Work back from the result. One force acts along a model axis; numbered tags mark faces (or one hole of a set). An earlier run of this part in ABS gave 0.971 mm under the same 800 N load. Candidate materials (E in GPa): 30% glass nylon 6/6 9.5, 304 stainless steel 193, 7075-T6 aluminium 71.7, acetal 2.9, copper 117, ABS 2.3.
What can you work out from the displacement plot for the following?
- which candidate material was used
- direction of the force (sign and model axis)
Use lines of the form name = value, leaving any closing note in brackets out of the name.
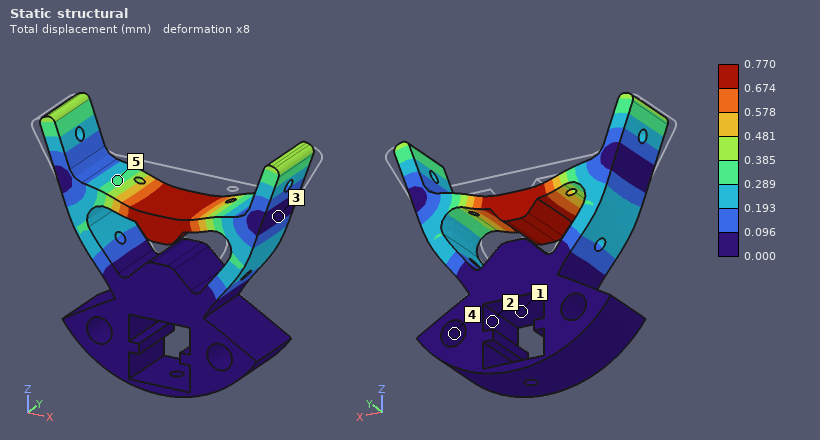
which candidate material was used = acetal
direction of the force = -Z
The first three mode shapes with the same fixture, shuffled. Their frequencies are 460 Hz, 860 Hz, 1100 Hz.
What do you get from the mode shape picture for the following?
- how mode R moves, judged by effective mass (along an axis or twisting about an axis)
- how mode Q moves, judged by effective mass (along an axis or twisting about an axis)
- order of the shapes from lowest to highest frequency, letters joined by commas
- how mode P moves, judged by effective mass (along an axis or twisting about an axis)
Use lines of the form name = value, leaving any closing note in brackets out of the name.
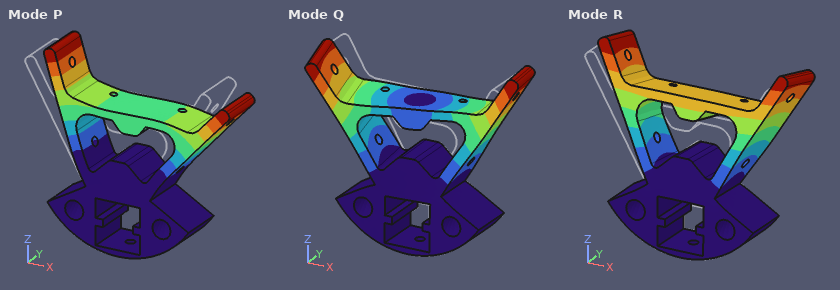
how mode R moves, judged by effective mass = along Y
how mode Q moves, judged by effective mass = twisting about Z
order of the shapes from lowest to highest frequency, letters joined by commas = P, R, Q
how mode P moves, judged by effective mass = along X
